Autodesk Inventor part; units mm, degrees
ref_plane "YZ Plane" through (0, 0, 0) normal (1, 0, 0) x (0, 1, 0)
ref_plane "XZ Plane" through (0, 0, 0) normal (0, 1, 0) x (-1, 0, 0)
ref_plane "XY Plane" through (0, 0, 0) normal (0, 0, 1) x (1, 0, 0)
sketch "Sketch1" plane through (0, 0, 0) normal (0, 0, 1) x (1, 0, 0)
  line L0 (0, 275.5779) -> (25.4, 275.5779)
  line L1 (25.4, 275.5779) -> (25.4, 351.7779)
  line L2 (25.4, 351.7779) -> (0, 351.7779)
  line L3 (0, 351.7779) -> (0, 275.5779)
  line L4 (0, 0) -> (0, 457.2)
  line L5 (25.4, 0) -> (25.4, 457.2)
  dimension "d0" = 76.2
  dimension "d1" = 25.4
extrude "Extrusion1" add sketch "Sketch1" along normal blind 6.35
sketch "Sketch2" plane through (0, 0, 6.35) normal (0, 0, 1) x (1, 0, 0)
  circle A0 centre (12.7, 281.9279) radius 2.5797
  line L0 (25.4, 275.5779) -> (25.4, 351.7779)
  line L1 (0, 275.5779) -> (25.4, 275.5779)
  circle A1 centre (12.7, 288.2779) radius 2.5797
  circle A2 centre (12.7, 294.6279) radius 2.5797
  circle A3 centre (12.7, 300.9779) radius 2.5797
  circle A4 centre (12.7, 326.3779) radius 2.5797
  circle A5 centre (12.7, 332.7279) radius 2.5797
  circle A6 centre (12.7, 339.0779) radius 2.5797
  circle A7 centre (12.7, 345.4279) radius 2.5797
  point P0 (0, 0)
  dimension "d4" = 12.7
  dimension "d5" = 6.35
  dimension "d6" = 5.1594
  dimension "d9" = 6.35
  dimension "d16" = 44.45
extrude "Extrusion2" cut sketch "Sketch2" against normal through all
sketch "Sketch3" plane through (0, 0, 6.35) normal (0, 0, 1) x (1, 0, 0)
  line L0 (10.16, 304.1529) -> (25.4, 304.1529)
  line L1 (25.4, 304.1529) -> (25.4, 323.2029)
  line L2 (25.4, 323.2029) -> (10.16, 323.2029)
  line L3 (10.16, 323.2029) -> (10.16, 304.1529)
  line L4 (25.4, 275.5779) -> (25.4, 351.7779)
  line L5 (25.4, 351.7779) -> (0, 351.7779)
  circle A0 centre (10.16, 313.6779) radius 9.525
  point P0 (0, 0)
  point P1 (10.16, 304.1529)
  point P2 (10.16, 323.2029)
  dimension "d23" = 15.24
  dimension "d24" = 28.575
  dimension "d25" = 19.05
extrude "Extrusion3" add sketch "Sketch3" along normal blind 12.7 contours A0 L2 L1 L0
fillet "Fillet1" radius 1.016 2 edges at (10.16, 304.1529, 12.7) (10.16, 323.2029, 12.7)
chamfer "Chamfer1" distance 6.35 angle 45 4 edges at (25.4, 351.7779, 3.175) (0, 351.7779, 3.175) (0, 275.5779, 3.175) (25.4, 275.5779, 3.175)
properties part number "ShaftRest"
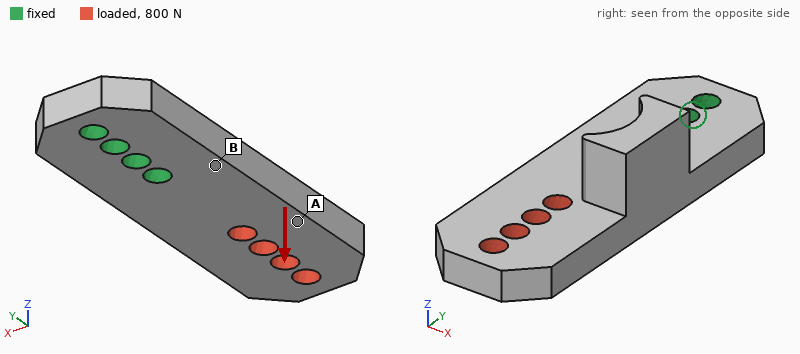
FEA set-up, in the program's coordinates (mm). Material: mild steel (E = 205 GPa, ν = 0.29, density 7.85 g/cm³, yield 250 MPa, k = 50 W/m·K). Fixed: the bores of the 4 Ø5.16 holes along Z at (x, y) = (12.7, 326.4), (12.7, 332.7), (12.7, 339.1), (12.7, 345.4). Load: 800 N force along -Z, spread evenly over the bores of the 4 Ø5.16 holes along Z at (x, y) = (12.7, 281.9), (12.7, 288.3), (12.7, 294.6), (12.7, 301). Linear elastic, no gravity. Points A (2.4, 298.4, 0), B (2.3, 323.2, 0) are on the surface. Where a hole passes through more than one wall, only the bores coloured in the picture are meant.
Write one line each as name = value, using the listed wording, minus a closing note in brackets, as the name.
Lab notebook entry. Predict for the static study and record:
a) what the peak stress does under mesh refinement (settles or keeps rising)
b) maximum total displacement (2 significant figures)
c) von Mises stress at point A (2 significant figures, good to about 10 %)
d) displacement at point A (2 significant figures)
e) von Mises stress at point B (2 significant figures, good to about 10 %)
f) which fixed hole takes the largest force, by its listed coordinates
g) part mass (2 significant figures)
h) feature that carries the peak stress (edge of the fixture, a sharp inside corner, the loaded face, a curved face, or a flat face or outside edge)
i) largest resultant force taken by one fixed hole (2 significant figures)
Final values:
what the peak stress does under mesh refinement = keeps rising
maximum total displacement = 0.15 mm
von Mises stress at point A = 36 MPa
displacement at point A = 0.060 mm
von Mises stress at point B = 80 MPa
which fixed hole takes the largest force, by its listed coordinates = (12.7, 326.4)
part mass = 98 g
feature that carries the peak stress = edge of the fixture
largest resultant force taken by one fixed hole = 1.8 kN
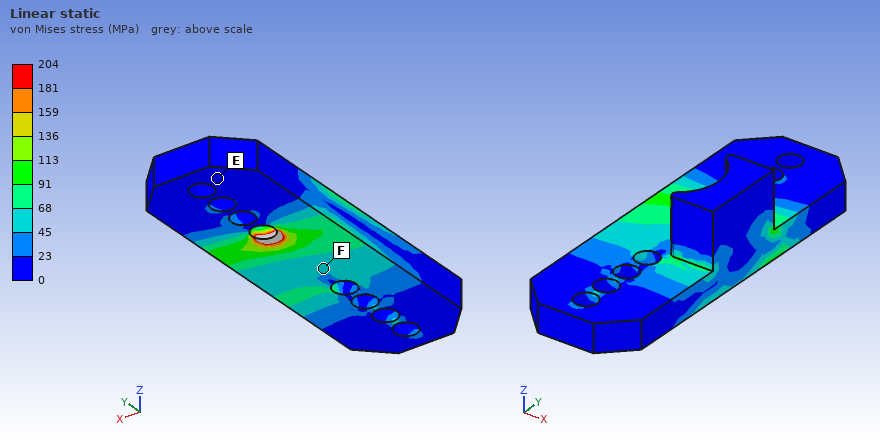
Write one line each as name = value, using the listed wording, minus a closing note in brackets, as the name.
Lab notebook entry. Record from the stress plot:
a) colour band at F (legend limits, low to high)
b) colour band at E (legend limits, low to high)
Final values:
colour band at F = 45 to 68 MPa
colour band at E = 0 to 23 MPa
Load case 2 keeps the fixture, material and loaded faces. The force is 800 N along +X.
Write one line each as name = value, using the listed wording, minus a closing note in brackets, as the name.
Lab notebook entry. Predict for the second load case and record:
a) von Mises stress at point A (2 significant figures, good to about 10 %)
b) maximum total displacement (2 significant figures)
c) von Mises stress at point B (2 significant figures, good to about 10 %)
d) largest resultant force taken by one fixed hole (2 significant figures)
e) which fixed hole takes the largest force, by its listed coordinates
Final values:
von Mises stress at point A = 9.5 MPa
maximum total displacement = 23 µm
von Mises stress at point B = 27 MPa
largest resultant force taken by one fixed hole = 2.0 kN
which fixed hole takes the largest force, by its listed coordinates = (12.7, 326.4)
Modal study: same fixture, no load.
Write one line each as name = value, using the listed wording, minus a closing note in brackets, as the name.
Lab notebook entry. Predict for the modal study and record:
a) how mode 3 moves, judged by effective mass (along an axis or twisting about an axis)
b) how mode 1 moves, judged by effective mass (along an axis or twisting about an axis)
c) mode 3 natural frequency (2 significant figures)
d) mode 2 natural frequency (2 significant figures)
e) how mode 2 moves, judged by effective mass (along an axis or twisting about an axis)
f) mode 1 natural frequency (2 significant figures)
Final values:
how mode 3 moves, judged by effective mass = twisting about Y
how mode 1 moves, judged by effective mass = along Z
mode 3 natural frequency = 6800 Hz
mode 2 natural frequency = 5800 Hz
how mode 2 moves, judged by effective mass = along X
mode 1 natural frequency = 2400 Hz
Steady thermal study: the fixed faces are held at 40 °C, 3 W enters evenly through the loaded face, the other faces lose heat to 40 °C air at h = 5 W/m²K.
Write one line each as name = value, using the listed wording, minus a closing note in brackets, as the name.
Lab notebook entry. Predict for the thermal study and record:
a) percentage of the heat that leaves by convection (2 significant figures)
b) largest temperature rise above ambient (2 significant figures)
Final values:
percentage of the heat that leaves by convection = 4.7 %
largest temperature rise above ambient = 14 K
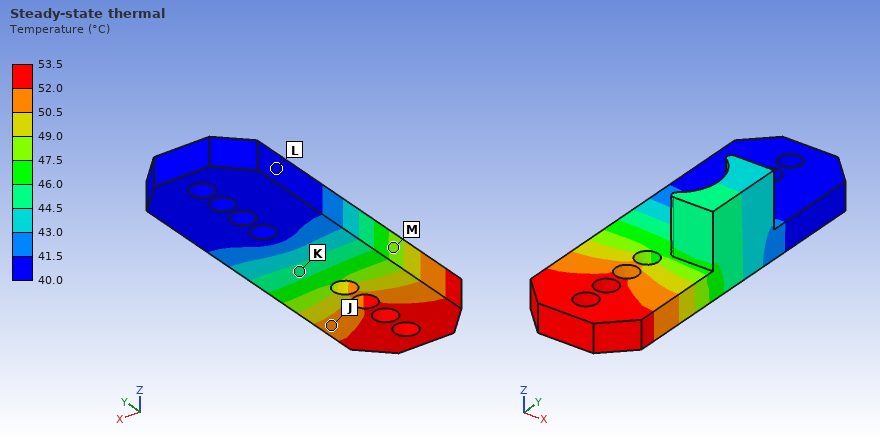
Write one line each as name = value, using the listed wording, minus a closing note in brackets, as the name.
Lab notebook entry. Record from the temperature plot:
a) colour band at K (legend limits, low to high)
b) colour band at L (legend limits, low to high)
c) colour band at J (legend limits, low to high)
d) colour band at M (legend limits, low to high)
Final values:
colour band at K = 44.5 to 46.0 °C
colour band at L = 40.0 to 41.5 °C
colour band at J = 50.5 to 52.0 °C
colour band at M = 47.5 to 49.0 °C
